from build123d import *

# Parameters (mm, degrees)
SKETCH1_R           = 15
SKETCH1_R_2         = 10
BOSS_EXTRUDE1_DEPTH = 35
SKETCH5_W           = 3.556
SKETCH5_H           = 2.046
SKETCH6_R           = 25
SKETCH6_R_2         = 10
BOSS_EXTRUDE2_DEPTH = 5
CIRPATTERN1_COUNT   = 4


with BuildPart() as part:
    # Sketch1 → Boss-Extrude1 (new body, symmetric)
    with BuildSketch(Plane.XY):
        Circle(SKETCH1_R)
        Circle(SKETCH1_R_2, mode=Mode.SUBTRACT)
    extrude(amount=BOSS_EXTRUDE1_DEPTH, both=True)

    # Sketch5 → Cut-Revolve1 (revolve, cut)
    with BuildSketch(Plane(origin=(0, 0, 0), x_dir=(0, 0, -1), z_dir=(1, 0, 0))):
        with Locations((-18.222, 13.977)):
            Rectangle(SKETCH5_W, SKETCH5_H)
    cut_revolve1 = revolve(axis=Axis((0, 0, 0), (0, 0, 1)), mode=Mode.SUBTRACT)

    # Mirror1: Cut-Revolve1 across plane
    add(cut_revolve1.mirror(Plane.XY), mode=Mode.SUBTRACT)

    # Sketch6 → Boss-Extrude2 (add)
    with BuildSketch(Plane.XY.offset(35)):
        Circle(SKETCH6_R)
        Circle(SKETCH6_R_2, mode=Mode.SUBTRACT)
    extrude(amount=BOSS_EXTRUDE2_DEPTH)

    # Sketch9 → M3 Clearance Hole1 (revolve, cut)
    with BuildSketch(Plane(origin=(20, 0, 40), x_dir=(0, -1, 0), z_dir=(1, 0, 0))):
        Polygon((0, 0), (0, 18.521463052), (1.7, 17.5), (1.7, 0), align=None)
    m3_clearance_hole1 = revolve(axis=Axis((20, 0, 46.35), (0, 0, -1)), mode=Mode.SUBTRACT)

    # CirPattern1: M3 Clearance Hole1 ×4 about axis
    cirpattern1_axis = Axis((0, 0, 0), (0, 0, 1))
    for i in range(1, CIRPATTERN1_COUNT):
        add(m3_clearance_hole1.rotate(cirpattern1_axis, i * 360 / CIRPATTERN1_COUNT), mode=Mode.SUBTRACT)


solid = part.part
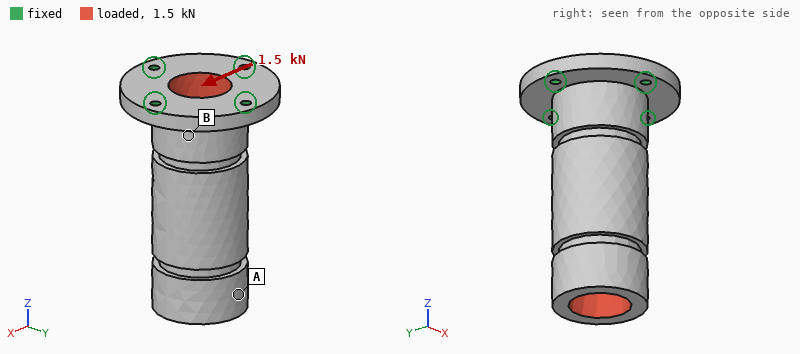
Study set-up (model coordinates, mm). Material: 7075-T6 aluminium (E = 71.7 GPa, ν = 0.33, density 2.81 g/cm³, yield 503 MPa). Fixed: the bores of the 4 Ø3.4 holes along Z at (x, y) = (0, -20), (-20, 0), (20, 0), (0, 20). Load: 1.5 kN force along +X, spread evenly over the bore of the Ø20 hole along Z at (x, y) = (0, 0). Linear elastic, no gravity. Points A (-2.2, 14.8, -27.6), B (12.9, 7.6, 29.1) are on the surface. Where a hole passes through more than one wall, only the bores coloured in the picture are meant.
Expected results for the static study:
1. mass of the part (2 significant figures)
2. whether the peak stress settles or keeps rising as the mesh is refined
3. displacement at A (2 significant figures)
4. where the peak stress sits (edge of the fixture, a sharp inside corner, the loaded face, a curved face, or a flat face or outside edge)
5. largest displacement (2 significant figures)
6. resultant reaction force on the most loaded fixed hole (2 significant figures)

96 g
keeps rising
78 µm
edge of the fixture
89 µm
1.5 kN
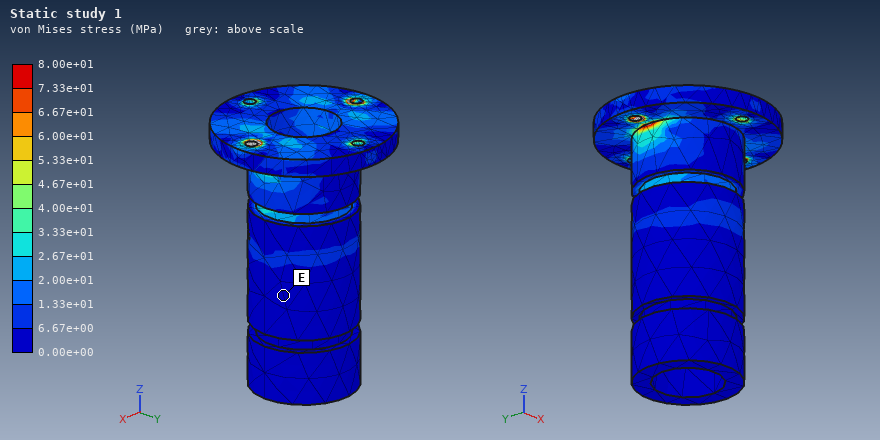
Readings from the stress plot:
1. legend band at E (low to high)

0.00e+00 to 6.67e+00 MPa
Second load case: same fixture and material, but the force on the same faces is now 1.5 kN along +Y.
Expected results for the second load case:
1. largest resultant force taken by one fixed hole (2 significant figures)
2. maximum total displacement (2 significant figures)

1.5 kN
90 µm
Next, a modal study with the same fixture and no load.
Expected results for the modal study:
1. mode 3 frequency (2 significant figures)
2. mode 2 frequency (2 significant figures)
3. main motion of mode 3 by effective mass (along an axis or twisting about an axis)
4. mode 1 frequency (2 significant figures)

9900 Hz
2800 Hz
twisting about Z
2800 Hz
